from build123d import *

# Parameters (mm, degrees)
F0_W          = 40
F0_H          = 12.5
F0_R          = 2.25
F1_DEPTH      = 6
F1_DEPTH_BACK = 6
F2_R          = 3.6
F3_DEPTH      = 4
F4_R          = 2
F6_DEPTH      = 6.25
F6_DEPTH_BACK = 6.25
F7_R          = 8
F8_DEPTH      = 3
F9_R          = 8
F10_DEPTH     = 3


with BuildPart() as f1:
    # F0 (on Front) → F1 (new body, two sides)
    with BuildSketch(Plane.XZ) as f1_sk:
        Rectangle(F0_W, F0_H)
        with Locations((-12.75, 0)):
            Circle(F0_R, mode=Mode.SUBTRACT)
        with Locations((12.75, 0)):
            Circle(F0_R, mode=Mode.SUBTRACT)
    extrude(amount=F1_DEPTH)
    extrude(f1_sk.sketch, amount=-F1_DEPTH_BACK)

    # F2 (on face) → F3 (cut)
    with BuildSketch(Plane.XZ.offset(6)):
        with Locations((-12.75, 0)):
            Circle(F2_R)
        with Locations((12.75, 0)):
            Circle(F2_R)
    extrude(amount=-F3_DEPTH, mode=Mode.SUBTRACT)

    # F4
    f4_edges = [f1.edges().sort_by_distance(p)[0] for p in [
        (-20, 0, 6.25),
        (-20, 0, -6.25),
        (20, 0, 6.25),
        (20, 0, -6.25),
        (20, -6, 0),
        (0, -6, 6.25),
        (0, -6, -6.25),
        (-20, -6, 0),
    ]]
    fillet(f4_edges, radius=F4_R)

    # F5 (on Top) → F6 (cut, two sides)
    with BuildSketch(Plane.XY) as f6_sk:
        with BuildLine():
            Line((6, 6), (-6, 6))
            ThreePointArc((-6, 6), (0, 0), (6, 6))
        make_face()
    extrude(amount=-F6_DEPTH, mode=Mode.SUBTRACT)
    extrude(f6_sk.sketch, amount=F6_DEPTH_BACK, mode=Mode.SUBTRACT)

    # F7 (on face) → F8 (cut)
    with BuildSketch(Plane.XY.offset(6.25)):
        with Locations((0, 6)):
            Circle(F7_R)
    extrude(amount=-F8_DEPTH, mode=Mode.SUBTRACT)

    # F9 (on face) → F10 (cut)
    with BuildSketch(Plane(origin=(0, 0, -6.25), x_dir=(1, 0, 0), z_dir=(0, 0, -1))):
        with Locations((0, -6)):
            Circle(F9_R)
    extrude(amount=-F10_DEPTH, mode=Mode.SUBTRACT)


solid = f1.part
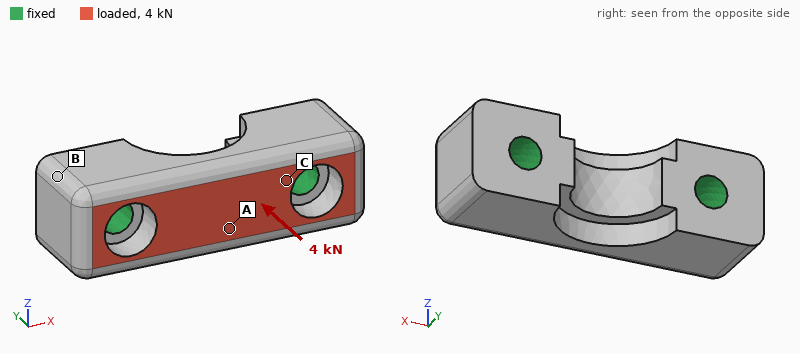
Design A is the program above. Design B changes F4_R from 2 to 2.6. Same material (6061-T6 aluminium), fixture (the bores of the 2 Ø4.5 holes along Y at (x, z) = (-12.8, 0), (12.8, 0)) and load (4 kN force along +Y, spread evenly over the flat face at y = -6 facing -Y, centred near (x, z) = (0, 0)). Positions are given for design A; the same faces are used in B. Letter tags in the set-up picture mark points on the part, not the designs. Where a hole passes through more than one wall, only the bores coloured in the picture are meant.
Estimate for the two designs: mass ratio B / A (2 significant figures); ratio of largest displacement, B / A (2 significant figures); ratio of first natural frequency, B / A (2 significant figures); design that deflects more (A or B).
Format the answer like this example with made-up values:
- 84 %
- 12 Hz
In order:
- 0.98
- 1.1
- 1.0
- B
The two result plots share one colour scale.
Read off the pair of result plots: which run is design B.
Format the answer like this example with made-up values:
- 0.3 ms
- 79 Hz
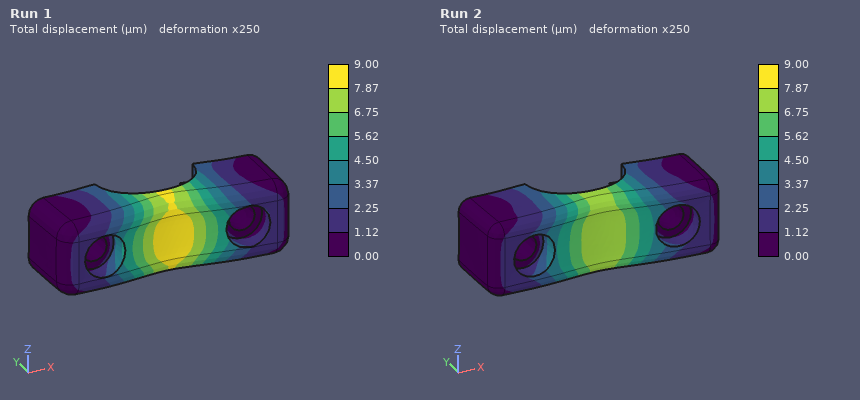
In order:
- Run 1
